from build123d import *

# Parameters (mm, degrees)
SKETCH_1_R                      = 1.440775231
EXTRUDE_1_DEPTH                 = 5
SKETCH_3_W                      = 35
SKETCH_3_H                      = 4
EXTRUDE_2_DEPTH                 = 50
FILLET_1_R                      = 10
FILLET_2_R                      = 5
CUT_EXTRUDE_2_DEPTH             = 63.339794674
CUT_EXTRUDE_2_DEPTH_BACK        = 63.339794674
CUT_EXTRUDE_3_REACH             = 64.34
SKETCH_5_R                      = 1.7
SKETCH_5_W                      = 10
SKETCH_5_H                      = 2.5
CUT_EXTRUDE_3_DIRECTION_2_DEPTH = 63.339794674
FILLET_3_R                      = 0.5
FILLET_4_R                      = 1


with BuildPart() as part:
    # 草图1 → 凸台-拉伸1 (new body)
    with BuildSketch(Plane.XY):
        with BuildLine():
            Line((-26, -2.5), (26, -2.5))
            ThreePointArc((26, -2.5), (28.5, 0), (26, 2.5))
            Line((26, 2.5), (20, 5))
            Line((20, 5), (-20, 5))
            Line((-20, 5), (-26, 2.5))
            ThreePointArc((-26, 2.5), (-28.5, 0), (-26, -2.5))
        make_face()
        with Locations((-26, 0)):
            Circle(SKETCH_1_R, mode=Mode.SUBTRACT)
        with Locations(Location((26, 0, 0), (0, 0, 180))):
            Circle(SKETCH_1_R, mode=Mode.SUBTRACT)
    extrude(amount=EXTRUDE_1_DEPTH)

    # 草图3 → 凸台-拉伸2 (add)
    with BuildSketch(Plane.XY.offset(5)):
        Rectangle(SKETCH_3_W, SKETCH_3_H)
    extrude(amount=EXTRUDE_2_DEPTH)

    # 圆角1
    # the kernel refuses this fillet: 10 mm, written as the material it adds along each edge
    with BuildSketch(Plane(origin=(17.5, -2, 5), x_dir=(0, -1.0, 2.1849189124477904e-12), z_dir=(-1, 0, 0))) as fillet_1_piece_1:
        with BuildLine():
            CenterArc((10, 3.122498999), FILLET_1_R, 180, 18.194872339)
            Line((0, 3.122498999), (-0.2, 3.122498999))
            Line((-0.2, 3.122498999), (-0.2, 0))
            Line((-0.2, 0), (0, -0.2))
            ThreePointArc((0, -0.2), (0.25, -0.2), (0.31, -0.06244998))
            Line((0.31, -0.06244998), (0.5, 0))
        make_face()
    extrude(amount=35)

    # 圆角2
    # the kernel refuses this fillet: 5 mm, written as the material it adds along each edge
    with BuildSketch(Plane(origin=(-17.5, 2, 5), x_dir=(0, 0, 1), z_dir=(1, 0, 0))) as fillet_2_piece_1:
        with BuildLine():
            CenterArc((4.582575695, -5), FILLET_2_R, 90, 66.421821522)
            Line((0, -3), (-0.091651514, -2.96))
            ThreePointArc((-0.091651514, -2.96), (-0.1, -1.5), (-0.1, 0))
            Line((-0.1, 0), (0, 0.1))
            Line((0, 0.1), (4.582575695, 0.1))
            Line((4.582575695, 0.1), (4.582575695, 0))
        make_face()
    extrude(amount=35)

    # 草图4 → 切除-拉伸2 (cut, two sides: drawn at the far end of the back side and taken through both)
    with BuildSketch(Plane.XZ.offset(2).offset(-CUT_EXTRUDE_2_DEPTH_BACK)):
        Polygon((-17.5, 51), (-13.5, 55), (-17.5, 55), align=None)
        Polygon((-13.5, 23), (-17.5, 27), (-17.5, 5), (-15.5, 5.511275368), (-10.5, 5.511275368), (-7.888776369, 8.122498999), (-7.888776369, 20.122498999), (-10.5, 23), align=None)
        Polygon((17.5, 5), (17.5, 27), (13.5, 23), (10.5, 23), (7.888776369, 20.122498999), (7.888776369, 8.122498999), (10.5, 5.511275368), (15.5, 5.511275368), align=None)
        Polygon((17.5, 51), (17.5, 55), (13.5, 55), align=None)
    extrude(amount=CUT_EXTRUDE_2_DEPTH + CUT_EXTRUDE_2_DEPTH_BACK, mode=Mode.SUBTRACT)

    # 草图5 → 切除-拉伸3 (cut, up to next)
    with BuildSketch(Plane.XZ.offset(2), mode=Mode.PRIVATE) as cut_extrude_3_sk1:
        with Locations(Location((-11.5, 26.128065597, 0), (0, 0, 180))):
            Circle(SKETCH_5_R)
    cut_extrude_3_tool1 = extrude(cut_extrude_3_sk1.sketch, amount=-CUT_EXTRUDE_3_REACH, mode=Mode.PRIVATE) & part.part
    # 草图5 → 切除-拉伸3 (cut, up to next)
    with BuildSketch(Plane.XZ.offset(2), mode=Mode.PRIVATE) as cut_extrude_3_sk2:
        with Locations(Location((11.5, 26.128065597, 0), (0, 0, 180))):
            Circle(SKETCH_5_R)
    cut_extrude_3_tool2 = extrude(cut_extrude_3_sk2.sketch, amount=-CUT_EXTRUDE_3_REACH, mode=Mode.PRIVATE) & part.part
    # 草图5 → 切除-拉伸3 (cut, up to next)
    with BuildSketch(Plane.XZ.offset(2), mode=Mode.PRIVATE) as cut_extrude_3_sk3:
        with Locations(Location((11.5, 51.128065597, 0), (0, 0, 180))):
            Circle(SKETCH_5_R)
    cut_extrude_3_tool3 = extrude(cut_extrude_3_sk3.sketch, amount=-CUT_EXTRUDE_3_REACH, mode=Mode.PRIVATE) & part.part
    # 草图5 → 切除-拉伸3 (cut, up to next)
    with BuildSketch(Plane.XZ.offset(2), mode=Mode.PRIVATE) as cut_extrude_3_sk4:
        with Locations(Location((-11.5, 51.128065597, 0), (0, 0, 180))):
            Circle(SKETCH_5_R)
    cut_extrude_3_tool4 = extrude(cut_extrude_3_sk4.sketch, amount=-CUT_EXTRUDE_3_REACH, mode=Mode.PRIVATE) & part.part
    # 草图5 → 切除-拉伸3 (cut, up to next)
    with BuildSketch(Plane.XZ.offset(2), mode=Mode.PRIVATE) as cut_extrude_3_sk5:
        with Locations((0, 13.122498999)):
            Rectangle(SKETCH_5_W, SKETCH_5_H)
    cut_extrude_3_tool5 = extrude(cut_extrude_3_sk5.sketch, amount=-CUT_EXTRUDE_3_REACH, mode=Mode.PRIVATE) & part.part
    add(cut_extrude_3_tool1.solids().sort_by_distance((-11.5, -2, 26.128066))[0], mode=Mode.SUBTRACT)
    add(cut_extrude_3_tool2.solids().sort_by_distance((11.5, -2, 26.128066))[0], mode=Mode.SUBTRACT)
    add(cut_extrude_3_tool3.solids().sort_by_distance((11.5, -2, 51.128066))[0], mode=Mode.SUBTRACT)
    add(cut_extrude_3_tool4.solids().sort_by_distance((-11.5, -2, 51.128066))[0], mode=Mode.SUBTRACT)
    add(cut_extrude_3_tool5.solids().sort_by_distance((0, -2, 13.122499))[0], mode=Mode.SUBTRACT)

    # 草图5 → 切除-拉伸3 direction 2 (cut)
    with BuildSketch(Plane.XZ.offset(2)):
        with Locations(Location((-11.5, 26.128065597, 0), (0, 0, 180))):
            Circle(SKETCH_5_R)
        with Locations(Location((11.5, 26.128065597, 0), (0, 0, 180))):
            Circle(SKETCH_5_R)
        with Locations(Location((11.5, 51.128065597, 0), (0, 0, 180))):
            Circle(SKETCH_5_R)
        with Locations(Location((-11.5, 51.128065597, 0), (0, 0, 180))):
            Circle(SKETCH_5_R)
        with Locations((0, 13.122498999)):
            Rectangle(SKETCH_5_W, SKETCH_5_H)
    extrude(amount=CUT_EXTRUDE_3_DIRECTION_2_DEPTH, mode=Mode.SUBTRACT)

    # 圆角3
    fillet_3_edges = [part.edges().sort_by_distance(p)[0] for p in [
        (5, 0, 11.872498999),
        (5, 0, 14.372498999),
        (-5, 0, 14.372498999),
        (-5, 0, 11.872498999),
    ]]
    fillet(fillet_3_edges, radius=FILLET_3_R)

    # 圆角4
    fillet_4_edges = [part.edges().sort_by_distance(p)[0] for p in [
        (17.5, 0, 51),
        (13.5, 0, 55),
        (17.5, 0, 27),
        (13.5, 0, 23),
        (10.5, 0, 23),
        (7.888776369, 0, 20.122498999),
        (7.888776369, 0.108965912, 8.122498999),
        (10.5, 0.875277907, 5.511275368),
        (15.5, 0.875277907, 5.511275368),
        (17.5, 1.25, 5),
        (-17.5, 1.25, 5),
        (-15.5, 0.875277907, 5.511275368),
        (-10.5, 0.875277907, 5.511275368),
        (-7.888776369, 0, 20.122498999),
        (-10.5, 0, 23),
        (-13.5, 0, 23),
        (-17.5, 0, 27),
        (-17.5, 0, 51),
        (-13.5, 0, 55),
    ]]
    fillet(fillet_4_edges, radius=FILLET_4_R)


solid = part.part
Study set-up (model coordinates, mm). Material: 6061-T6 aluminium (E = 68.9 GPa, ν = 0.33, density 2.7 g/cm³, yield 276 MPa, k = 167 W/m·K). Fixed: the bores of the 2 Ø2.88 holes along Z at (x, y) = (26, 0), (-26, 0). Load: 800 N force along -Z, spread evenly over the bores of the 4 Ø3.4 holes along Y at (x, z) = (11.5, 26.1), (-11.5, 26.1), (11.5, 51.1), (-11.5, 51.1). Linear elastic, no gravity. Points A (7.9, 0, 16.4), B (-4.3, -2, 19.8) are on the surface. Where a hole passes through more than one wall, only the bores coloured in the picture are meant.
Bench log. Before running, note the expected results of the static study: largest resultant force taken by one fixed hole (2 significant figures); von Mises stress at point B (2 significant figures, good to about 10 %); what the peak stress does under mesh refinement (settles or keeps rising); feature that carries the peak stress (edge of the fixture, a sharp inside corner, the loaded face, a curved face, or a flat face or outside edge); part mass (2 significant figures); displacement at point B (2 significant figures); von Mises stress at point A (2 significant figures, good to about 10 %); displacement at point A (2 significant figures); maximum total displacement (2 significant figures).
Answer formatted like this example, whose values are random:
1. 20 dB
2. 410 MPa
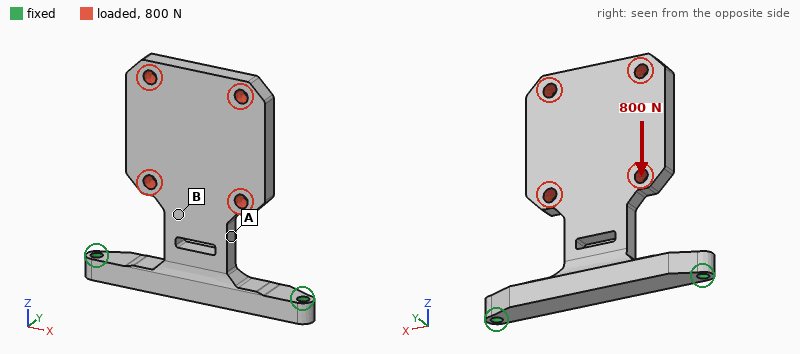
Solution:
1. 490 N
2. 11 MPa
3. keeps rising
4. edge of the fixture
5. 20 g
6. 64 µm
7. 24 MPa
8. 58 µm
9. 100 µm
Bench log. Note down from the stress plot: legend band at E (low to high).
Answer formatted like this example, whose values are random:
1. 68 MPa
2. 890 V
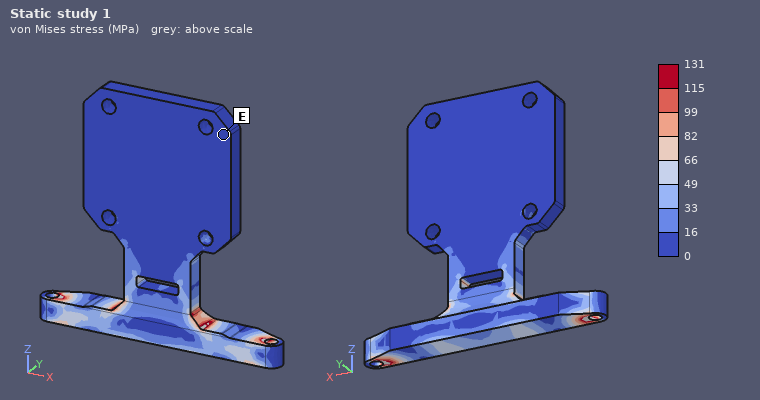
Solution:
1. 0 to 16 MPa
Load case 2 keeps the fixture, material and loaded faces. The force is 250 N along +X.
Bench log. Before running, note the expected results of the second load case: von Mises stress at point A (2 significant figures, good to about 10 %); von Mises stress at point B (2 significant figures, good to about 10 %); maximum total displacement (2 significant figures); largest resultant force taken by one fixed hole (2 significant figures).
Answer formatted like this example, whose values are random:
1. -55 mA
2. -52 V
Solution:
1. 27 MPa
2. 15 MPa
3. 0.15 mm
4. 270 N
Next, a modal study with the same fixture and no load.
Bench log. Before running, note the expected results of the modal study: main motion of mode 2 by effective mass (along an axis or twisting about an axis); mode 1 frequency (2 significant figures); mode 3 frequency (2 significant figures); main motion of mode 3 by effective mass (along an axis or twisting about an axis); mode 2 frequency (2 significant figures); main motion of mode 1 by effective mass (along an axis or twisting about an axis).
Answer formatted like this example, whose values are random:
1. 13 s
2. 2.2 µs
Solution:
1. along X
2. 580 Hz
3. 2600 Hz
4. twisting about Z
5. 2200 Hz
6. along Y
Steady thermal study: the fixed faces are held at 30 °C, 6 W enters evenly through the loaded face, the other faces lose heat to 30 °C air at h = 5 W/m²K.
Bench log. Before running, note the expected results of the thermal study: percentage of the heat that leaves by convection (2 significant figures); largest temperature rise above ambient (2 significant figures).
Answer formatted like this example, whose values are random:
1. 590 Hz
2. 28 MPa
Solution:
1. 7.2 %
2. 29 K
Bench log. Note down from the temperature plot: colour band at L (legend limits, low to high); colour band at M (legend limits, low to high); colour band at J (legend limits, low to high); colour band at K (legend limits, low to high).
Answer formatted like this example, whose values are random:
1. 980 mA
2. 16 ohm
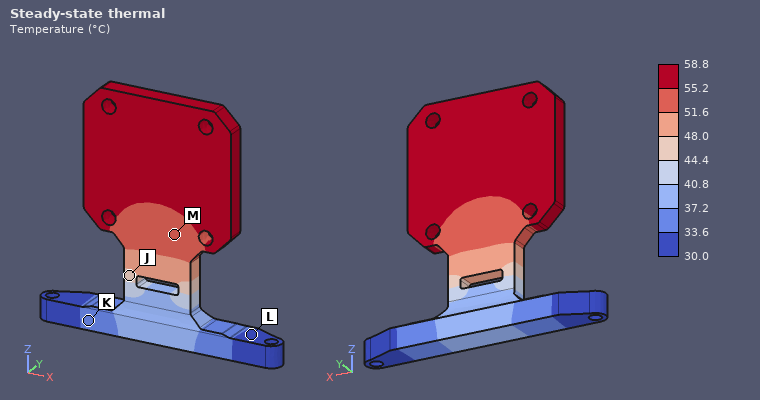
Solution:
1. 30.0 to 33.6 °C
2. 51.6 to 55.2 °C
3. 44.4 to 48.0 °C
4. 33.6 to 37.2 °C
